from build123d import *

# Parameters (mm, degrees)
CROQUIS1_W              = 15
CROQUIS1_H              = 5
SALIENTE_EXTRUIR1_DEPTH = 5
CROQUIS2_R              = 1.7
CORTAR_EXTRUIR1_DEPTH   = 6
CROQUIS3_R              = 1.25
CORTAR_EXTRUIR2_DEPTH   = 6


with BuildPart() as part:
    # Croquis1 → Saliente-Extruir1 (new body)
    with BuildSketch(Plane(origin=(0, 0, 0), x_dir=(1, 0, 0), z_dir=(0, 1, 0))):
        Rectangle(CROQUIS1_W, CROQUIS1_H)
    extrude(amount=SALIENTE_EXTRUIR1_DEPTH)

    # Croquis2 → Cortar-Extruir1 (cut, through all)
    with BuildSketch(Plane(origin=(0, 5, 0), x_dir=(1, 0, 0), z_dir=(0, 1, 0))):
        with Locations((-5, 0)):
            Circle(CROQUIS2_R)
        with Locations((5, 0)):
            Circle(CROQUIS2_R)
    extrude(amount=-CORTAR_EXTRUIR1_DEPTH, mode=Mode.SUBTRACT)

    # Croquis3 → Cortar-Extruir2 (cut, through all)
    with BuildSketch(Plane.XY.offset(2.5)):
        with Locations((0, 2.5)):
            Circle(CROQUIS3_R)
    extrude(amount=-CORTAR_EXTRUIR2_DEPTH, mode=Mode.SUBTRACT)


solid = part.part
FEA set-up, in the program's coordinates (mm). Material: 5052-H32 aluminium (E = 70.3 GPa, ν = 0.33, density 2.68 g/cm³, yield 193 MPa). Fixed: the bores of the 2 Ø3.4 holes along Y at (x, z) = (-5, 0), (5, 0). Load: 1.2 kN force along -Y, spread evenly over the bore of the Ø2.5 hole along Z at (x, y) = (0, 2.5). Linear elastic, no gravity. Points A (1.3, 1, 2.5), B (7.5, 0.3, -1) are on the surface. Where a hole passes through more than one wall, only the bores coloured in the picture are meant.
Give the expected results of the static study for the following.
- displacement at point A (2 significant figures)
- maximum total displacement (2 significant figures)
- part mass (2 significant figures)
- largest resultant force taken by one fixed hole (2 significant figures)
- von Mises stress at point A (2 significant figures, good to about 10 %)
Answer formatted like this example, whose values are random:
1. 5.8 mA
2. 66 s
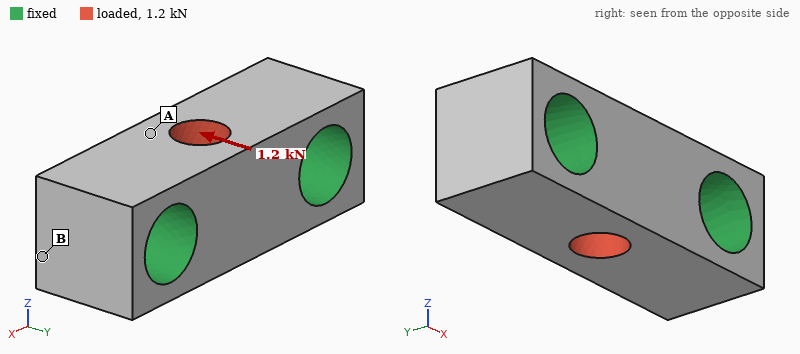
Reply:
1. 3.0 µm
2. 4.5 µm
3. 0.70 g
4. 600 N
5. 44 MPa
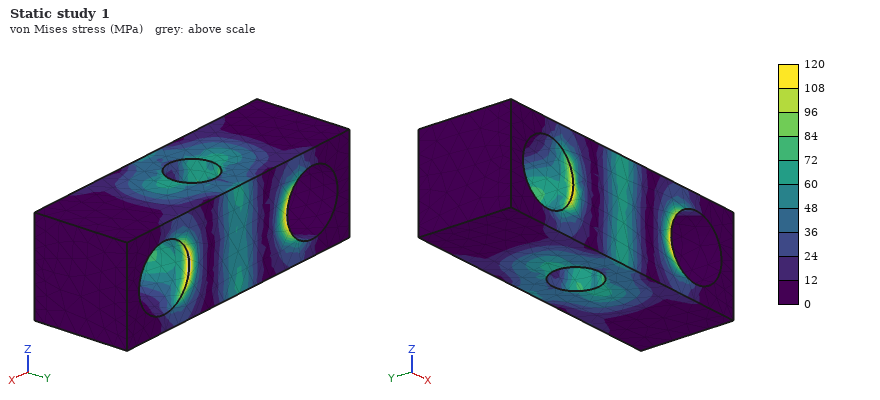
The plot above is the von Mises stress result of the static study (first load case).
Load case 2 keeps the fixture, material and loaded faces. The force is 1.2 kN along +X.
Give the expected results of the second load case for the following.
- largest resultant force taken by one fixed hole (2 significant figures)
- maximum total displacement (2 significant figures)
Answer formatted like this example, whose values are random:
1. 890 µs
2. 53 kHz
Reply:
1. 600 N
2. 1.4 µm
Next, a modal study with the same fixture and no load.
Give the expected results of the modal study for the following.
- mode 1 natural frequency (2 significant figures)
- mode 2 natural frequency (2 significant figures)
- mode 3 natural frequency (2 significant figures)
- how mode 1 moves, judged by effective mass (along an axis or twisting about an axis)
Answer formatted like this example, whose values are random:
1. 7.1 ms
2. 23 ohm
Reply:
1. 190 kHz
2. 200 kHz
3. 210 kHz
4. along Z
